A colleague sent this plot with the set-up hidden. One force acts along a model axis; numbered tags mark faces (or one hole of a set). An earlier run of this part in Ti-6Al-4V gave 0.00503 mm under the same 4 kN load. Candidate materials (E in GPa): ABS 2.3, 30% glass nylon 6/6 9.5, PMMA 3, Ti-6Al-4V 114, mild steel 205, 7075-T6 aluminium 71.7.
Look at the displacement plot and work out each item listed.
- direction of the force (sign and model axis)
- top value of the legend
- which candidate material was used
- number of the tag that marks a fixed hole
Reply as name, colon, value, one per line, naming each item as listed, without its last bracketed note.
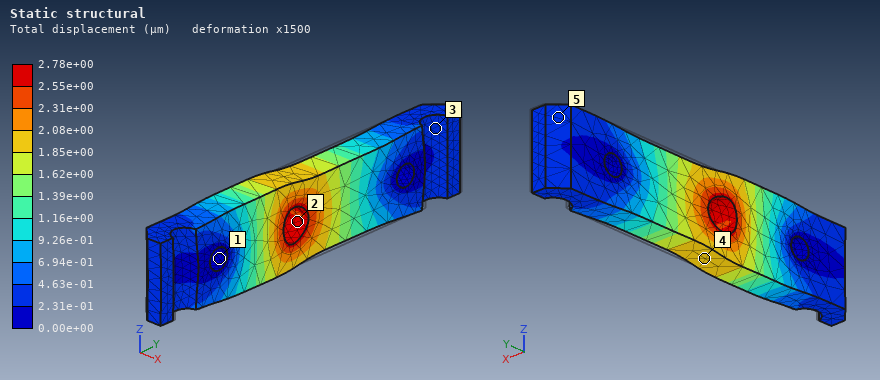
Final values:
direction of the force: -Y
top value of the legend: 2.78e+00 µm
which candidate material was used: mild steel
number of the tag that marks a fixed hole: 1
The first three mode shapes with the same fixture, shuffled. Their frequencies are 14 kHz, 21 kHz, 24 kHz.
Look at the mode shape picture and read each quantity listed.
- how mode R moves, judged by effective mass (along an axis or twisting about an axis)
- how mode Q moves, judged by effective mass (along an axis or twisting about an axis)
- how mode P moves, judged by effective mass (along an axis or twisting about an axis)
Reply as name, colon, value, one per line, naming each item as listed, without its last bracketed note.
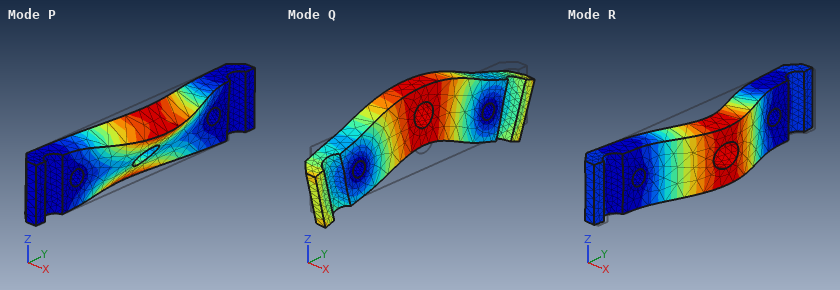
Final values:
how mode R moves, judged by effective mass: along X
how mode Q moves, judged by effective mass: along Z
how mode P moves, judged by effective mass: twisting about Y
